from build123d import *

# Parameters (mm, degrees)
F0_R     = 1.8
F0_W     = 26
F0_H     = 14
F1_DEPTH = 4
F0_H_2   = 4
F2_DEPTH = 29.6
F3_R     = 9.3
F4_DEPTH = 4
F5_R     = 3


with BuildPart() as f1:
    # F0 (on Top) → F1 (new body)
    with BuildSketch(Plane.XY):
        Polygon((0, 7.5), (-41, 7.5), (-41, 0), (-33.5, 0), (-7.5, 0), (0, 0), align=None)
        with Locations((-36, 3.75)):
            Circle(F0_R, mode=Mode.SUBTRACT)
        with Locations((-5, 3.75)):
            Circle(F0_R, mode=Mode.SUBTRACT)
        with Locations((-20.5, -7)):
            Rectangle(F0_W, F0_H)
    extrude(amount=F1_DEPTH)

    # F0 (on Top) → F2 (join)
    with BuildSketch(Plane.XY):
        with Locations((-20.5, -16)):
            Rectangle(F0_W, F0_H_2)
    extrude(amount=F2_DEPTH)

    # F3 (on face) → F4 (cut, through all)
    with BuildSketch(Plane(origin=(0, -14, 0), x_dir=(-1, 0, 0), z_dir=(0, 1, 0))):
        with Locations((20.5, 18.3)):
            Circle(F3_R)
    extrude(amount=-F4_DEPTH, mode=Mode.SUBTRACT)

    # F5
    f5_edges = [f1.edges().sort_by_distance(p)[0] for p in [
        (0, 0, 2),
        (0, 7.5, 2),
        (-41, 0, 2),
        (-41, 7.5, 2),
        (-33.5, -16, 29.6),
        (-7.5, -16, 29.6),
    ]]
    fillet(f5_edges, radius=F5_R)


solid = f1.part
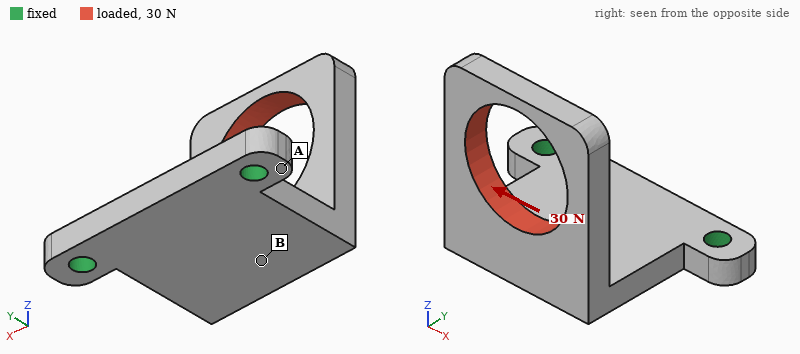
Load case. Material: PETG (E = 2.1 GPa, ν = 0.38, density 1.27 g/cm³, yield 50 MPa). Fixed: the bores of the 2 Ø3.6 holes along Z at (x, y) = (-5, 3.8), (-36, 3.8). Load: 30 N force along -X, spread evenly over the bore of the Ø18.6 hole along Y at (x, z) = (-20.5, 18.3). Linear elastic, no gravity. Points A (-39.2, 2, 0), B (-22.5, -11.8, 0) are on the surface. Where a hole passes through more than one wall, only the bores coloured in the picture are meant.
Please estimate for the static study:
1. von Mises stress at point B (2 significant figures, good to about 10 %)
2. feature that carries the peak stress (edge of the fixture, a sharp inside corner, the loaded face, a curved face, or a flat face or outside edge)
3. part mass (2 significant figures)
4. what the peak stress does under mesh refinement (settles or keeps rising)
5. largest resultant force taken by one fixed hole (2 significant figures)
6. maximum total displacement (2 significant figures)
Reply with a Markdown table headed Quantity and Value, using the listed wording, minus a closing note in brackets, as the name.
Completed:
| Quantity | Value |
|---|---|
| von Mises stress at point B | 3.3 MPa |
| feature that carries the peak stress | edge of the fixture |
| part mass | 5.8 g |
| what the peak stress does under mesh refinement | keeps rising |
| largest resultant force taken by one fixed hole | 33 N |
| maximum total displacement | 0.53 mm |
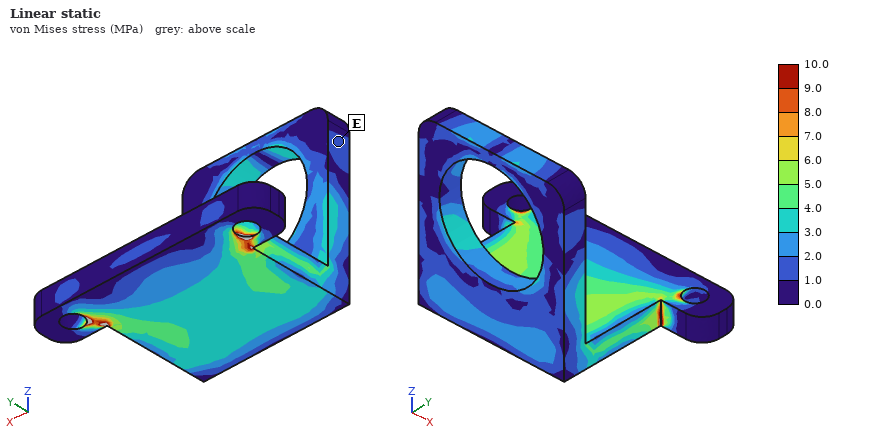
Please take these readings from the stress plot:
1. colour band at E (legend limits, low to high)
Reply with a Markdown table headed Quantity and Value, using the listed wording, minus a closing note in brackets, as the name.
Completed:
| Quantity | Value |
|---|---|
| colour band at E | 1.0 to 2.0 MPa |
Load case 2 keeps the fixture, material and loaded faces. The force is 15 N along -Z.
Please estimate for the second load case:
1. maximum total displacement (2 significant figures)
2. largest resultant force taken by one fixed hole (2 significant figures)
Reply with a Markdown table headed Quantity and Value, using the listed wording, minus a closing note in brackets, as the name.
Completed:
| Quantity | Value |
|---|---|
| maximum total displacement | 0.51 mm |
| largest resultant force taken by one fixed hole | 7.5 N |
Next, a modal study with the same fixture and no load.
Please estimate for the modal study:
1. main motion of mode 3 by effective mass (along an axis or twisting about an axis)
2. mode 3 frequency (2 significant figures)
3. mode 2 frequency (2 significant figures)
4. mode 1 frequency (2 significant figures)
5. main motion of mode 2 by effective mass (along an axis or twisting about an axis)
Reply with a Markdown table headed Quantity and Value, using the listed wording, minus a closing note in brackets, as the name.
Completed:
| Quantity | Value |
|---|---|
| main motion of mode 3 by effective mass | along Z |
| mode 3 frequency | 1300 Hz |
| mode 2 frequency | 1000 Hz |
| mode 1 frequency | 510 Hz |
| main motion of mode 2 by effective mass | along X |
